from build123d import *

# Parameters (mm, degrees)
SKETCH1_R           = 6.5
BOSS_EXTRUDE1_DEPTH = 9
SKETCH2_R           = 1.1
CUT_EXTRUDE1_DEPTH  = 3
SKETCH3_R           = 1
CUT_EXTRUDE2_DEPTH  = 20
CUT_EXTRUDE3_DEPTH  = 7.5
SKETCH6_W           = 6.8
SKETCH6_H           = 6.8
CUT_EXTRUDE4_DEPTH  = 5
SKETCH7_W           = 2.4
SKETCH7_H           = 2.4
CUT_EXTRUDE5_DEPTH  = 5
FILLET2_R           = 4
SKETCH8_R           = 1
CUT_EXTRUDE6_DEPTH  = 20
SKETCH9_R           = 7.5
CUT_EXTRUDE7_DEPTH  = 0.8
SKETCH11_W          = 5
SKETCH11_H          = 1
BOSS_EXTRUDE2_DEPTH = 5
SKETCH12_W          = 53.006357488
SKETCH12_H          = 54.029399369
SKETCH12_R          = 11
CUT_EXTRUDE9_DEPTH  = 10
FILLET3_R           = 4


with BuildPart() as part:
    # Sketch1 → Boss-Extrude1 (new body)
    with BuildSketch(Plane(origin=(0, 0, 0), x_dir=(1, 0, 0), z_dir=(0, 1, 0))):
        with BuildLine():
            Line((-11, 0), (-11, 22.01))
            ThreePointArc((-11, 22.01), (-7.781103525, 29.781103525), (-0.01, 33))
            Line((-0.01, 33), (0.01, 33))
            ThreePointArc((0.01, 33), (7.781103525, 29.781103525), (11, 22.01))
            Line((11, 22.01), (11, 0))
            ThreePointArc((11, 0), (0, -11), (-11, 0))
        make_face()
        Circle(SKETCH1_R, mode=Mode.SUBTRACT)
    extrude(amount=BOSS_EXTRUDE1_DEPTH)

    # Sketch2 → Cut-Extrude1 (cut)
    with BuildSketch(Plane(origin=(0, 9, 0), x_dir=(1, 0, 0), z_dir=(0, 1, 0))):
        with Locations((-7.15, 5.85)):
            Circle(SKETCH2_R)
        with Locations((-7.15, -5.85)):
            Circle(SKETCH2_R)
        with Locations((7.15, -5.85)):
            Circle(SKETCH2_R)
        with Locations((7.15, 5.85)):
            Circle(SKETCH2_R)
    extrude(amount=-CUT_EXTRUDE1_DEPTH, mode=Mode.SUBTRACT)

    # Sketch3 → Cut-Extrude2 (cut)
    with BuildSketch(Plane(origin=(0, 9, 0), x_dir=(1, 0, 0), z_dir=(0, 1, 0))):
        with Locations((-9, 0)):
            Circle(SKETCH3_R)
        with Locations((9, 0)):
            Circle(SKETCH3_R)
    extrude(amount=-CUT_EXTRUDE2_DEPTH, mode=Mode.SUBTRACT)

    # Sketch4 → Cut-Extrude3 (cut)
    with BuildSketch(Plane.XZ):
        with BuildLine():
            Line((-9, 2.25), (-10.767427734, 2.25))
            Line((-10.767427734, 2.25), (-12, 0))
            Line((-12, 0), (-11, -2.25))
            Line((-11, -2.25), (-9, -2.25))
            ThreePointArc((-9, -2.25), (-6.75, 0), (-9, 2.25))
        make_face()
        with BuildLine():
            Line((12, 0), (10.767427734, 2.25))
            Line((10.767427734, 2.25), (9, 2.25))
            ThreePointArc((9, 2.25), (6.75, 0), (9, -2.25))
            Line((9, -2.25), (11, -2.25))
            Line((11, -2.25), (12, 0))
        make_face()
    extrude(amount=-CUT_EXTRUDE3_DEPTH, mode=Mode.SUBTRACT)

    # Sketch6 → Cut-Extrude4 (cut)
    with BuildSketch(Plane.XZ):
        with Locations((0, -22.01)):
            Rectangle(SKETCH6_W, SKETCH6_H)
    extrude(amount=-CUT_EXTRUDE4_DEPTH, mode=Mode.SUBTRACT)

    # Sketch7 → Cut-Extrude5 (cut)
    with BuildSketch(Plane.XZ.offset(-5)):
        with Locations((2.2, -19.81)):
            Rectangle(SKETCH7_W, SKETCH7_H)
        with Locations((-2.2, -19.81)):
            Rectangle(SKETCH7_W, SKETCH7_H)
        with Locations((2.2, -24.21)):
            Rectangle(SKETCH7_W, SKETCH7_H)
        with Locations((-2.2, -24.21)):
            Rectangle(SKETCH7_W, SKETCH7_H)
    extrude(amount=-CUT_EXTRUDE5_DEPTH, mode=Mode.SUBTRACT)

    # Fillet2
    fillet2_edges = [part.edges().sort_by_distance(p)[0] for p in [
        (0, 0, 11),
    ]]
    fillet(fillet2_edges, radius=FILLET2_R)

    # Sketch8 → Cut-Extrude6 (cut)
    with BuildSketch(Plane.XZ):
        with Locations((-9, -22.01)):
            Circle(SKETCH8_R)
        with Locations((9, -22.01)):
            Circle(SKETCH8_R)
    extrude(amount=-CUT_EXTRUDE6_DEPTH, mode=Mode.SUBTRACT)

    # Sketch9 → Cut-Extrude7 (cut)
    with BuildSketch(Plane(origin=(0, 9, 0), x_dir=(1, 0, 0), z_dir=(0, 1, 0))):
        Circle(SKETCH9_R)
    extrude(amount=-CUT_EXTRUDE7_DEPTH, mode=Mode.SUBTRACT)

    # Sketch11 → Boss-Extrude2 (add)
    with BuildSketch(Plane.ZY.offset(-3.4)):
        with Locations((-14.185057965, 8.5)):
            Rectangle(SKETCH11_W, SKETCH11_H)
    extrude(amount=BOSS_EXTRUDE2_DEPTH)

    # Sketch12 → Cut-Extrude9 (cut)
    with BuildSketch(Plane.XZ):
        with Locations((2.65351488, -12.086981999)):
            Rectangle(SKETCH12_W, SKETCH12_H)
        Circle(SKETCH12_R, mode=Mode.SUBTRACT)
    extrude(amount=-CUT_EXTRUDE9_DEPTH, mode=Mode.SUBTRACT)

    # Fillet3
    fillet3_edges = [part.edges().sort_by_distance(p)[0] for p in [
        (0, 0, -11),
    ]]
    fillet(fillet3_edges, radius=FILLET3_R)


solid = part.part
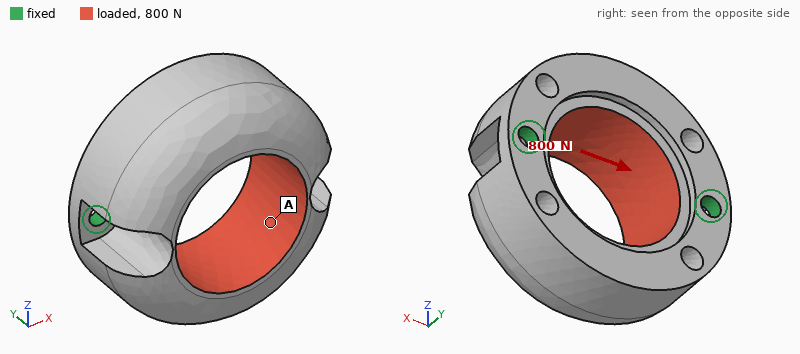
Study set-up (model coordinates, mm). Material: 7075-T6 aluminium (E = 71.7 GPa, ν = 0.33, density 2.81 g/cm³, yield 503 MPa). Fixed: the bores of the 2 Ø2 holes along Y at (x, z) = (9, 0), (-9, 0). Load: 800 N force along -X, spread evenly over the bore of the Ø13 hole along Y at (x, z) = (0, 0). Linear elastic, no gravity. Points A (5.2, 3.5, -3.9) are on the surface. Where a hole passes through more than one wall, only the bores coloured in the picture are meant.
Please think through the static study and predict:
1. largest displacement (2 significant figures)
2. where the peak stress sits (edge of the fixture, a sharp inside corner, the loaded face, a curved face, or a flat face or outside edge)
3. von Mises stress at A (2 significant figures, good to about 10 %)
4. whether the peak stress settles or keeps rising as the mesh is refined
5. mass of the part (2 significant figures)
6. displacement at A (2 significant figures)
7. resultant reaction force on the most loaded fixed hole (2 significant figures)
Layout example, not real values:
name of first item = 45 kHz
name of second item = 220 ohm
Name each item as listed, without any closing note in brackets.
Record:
largest displacement = 13 µm
where the peak stress sits = edge of the fixture
von Mises stress at A = 21 MPa
whether the peak stress settles or keeps rising as the mesh is refined = keeps rising
mass of the part = 4.8 g
displacement at A = 8.2 µm
resultant reaction force on the most loaded fixed hole = 440 N
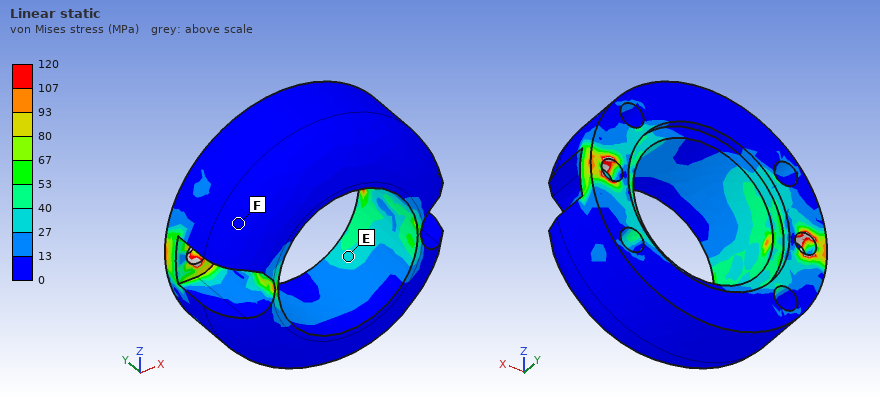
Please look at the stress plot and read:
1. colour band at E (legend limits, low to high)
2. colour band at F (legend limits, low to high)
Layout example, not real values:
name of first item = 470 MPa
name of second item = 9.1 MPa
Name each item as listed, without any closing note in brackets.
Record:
colour band at E = 27 to 40 MPa
colour band at F = 0 to 13 MPa
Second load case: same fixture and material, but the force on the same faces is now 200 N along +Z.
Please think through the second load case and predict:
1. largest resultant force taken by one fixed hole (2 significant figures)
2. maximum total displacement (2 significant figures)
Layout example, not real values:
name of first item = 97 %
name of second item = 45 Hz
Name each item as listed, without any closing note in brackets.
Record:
largest resultant force taken by one fixed hole = 100 N
maximum total displacement = 29 µm
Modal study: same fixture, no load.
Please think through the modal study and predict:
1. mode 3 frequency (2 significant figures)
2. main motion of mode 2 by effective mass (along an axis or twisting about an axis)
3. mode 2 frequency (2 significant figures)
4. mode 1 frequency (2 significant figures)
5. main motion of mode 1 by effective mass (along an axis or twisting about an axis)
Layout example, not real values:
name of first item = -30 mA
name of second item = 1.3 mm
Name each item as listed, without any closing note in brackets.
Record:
mode 3 frequency = 23 kHz
main motion of mode 2 by effective mass = along Y
mode 2 frequency = 21 kHz
mode 1 frequency = 5800 Hz
main motion of mode 1 by effective mass = along Z
